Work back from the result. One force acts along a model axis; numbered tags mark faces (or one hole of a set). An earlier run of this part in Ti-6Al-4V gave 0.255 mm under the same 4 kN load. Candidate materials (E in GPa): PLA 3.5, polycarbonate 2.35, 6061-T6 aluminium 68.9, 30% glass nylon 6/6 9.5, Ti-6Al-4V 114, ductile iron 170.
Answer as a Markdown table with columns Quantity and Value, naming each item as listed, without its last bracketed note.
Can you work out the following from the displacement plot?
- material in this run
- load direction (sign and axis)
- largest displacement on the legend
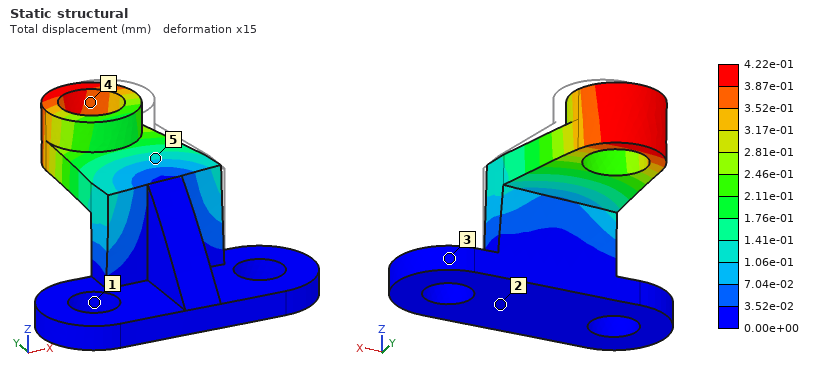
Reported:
| Quantity | Value |
|---|---|
| material in this run | 6061-T6 aluminium |
| load direction | -X |
| largest displacement on the legend | 4.22e-01 mm |
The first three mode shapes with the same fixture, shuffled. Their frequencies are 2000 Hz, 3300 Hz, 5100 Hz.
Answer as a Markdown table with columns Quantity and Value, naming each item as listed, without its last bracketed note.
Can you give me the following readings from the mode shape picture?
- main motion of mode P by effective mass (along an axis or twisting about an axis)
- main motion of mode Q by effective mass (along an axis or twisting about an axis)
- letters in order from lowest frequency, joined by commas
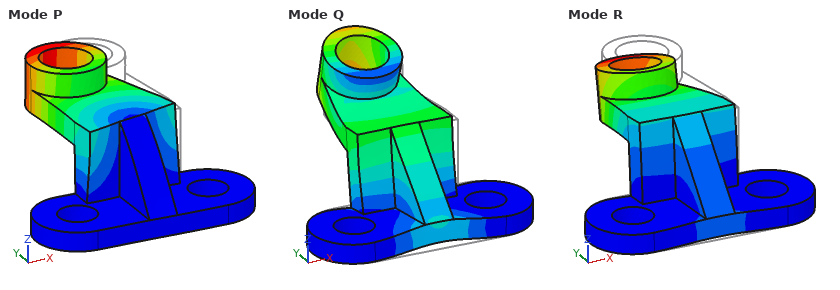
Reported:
| Quantity | Value |
|---|---|
| main motion of mode P by effective mass | along X |
| main motion of mode Q by effective mass | along Y |
| letters in order from lowest frequency, joined by commas | R, P, Q |
